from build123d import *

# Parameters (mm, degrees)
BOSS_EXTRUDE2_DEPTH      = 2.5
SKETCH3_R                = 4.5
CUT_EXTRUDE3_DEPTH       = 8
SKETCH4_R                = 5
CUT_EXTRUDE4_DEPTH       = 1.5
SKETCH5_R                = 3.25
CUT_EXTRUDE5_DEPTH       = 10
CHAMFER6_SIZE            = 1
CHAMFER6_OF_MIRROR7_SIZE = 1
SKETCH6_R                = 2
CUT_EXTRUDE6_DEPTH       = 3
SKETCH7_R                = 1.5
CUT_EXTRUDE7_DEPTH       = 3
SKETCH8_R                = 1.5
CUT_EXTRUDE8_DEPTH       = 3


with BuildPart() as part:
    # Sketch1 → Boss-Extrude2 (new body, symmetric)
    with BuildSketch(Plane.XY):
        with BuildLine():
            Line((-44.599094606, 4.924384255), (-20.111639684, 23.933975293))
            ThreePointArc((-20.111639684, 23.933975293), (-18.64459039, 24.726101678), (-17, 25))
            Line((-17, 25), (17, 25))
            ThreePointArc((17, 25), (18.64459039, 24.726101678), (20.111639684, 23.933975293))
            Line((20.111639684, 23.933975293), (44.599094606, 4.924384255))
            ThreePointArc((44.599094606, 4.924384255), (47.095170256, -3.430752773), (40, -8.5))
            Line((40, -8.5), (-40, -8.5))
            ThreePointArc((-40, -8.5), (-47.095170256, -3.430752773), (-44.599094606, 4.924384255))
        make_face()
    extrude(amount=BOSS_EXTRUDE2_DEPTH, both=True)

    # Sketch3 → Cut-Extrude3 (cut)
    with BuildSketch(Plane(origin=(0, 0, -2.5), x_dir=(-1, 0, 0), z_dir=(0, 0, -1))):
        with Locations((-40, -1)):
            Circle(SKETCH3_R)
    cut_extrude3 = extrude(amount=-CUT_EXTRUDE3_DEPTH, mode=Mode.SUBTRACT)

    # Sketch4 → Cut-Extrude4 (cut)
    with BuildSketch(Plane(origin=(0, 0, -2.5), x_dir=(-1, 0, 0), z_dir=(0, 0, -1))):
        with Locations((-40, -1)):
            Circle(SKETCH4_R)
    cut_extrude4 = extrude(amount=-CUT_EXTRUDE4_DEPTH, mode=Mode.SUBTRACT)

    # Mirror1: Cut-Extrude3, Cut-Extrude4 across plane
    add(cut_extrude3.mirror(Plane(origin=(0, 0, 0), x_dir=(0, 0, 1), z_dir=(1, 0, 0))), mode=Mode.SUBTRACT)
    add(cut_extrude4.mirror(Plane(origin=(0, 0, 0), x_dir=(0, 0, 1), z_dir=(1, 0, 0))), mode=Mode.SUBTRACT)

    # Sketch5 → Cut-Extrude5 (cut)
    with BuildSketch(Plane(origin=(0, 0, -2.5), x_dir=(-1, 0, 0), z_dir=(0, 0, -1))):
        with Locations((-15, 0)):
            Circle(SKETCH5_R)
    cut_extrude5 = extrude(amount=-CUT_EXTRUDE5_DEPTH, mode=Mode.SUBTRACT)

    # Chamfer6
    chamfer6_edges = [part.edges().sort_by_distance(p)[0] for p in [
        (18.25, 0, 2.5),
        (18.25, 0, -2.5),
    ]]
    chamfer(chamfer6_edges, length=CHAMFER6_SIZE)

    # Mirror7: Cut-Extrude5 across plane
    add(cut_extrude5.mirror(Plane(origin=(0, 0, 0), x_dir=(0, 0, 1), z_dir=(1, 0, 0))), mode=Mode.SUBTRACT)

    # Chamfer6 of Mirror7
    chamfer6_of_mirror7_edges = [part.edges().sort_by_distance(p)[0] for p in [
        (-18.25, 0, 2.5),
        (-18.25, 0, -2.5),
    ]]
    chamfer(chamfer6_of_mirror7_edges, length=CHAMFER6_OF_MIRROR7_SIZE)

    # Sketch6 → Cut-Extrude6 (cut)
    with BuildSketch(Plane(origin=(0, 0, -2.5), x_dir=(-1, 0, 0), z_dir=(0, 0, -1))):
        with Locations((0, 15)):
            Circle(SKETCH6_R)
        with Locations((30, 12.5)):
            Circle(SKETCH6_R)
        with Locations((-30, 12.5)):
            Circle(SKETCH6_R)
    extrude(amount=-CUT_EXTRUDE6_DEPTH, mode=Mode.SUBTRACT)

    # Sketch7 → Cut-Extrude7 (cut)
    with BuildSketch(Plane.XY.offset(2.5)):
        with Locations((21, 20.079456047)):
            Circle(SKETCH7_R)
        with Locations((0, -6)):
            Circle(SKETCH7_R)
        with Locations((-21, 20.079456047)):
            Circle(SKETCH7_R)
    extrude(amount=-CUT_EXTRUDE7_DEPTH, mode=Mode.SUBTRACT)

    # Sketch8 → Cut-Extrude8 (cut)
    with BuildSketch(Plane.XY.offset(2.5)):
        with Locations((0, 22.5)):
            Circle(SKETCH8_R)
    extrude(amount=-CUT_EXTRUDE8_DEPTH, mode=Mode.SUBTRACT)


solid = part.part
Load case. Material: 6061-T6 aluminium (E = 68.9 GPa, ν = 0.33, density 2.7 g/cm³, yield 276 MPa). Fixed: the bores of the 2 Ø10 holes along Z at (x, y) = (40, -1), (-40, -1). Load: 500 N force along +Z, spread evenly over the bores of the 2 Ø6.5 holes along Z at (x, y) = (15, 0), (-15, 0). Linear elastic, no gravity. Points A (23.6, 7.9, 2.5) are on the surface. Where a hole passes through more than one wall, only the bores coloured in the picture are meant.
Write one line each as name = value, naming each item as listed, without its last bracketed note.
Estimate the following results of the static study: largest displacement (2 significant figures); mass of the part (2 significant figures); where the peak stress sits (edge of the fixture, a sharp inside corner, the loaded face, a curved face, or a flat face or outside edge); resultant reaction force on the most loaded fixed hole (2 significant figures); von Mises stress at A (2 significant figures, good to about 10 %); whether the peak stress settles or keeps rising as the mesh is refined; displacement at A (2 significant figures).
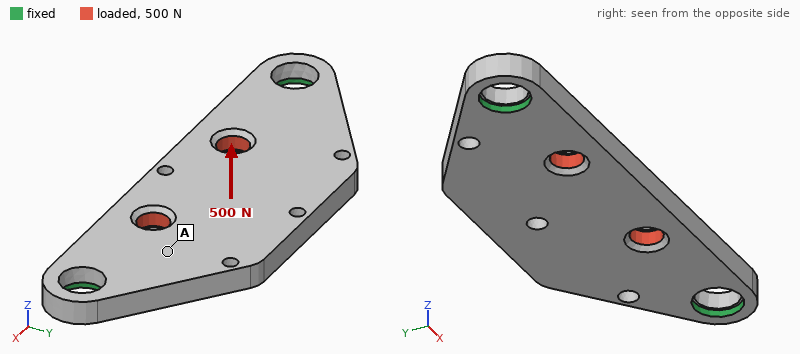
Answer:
largest displacement = 64 µm
mass of the part = 31 g
where the peak stress sits = edge of the fixture
resultant reaction force on the most loaded fixed hole = 340 N
von Mises stress at A = 12 MPa
whether the peak stress settles or keeps rising as the mesh is refined = keeps rising
displacement at A = 25 µm
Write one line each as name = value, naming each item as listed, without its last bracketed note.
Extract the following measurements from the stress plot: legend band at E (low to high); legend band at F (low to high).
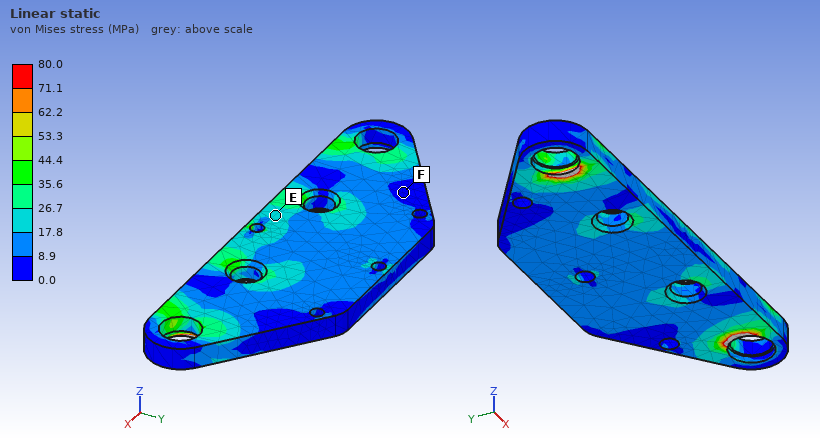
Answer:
legend band at E = 17.8 to 26.7 MPa
legend band at F = 0.0 to 8.9 MPa
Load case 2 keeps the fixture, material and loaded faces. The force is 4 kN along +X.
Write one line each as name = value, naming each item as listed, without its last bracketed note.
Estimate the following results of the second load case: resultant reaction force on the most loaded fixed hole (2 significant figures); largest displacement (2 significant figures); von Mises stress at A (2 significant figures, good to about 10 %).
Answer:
resultant reaction force on the most loaded fixed hole = 2.0 kN
largest displacement = 13 µm
von Mises stress at A = 9.6 MPa
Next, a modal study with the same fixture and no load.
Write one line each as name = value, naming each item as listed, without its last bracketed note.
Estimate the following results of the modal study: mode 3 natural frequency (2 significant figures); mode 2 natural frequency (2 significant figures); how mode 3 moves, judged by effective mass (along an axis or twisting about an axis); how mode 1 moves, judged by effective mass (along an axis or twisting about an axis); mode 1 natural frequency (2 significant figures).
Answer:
mode 3 natural frequency = 8000 Hz
mode 2 natural frequency = 5500 Hz
how mode 3 moves, judged by effective mass = twisting about Y
how mode 1 moves, judged by effective mass = along Z
mode 1 natural frequency = 2900 Hz
